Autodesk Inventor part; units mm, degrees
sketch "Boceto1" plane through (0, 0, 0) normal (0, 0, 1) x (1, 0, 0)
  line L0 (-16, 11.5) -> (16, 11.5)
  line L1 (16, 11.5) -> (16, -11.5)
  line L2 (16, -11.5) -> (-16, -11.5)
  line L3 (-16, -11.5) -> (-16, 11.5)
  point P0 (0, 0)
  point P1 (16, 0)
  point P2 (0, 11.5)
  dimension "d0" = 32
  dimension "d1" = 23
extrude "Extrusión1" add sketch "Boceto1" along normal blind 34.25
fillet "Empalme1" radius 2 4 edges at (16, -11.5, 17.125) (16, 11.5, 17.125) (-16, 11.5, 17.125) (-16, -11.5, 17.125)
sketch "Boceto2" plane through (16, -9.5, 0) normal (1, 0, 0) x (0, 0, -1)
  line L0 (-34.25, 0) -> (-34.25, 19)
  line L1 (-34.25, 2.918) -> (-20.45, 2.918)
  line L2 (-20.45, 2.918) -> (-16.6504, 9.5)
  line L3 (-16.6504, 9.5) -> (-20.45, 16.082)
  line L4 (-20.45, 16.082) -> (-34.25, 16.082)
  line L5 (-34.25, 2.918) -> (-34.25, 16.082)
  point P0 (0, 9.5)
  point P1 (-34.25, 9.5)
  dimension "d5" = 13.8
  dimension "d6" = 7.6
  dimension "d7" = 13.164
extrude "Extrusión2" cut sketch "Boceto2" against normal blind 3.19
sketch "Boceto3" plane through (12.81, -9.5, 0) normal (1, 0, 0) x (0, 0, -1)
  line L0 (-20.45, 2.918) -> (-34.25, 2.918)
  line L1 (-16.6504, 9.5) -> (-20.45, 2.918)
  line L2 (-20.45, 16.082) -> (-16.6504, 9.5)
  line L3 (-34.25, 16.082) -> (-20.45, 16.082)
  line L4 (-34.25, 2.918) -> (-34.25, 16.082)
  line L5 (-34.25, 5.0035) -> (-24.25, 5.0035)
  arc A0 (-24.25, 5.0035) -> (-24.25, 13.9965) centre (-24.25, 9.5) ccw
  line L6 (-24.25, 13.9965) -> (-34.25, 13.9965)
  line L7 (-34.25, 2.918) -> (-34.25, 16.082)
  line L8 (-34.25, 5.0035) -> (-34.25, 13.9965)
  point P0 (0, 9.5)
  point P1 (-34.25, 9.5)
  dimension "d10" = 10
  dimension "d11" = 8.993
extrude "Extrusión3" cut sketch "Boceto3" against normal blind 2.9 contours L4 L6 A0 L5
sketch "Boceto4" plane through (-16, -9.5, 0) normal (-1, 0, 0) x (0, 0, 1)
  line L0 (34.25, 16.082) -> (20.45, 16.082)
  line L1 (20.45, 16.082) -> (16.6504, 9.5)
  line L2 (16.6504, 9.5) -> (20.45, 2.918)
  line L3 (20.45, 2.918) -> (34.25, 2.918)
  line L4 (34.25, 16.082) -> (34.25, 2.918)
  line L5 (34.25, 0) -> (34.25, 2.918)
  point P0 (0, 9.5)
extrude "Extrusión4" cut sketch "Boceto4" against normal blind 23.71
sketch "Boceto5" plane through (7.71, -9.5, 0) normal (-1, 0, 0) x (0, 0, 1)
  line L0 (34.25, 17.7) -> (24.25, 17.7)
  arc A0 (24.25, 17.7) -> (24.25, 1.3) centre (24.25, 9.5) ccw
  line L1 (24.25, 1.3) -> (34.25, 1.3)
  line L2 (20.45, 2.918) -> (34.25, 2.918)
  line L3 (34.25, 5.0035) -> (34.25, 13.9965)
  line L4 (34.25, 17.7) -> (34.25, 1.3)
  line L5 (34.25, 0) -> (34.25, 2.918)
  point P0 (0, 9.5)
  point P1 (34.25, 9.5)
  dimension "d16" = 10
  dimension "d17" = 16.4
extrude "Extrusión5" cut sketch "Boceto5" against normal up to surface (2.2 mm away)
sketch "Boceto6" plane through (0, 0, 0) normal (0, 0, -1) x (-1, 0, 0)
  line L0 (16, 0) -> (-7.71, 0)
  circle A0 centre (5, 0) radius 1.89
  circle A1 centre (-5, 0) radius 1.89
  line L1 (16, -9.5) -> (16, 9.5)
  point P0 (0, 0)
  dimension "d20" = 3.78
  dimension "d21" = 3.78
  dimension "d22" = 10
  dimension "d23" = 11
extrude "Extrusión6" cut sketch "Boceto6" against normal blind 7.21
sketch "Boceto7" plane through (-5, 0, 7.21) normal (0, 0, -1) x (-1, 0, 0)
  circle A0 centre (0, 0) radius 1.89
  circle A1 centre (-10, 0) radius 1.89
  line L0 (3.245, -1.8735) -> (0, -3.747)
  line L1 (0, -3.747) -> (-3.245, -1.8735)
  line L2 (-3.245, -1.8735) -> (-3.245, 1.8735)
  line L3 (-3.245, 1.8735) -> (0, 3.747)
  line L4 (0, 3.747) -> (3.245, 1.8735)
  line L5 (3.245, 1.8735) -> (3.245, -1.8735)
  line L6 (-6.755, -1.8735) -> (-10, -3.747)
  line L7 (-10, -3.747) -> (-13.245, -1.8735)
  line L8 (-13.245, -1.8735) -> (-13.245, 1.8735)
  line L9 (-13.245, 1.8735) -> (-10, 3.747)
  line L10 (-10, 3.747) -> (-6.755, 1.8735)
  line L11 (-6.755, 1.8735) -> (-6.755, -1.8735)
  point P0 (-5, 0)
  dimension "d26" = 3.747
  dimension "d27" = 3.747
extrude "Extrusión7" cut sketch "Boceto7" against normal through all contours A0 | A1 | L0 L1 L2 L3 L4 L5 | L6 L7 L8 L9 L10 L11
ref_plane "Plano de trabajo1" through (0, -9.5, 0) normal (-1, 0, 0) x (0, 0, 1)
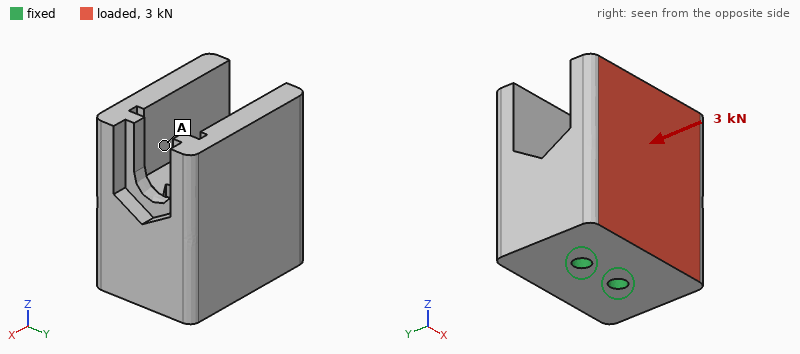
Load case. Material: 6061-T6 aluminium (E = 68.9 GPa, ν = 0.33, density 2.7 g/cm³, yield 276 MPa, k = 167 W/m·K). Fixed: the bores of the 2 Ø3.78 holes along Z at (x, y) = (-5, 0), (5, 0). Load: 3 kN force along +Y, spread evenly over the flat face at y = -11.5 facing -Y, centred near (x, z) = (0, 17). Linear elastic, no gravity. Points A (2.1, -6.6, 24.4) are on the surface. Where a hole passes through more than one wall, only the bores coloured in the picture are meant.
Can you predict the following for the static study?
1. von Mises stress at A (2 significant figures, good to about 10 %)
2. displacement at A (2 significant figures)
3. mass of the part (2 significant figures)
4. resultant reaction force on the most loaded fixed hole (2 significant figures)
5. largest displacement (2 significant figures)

26 MPa
0.055 mm
48 g
1.5 kN
0.11 mm
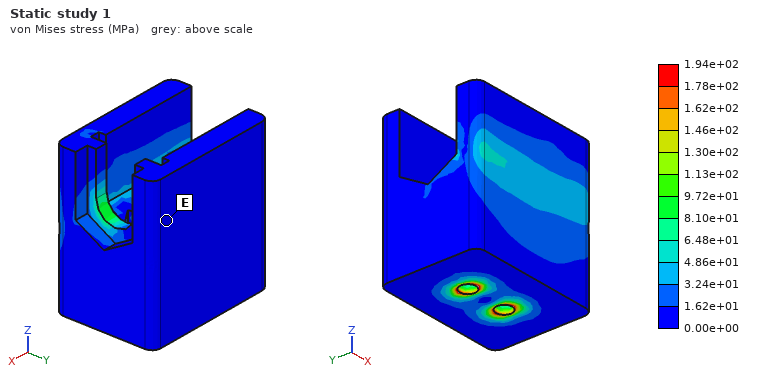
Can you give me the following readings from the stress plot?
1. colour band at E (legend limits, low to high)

0.00e+00 to 1.62e+01 MPa
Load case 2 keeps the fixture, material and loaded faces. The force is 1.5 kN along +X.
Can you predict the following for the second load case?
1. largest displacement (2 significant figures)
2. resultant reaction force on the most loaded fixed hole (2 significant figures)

22 µm
1.9 kN
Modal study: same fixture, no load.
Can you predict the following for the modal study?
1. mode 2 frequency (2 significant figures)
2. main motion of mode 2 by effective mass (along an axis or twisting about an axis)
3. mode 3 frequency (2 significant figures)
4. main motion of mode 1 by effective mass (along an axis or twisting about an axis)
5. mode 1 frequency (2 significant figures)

9600 Hz
along X
13 kHz
along Y
6500 Hz
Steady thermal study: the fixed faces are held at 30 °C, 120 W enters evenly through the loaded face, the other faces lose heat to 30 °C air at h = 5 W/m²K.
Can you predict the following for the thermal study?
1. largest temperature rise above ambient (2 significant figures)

49 K
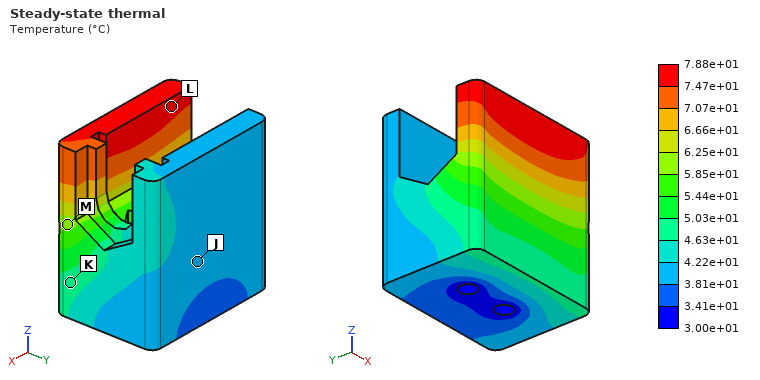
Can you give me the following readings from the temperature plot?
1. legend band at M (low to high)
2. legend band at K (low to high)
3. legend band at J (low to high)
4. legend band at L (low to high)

5.85e+01 to 6.25e+01 °C
4.63e+01 to 5.03e+01 °C
3.81e+01 to 4.22e+01 °C
7.47e+01 to 7.88e+01 °C
